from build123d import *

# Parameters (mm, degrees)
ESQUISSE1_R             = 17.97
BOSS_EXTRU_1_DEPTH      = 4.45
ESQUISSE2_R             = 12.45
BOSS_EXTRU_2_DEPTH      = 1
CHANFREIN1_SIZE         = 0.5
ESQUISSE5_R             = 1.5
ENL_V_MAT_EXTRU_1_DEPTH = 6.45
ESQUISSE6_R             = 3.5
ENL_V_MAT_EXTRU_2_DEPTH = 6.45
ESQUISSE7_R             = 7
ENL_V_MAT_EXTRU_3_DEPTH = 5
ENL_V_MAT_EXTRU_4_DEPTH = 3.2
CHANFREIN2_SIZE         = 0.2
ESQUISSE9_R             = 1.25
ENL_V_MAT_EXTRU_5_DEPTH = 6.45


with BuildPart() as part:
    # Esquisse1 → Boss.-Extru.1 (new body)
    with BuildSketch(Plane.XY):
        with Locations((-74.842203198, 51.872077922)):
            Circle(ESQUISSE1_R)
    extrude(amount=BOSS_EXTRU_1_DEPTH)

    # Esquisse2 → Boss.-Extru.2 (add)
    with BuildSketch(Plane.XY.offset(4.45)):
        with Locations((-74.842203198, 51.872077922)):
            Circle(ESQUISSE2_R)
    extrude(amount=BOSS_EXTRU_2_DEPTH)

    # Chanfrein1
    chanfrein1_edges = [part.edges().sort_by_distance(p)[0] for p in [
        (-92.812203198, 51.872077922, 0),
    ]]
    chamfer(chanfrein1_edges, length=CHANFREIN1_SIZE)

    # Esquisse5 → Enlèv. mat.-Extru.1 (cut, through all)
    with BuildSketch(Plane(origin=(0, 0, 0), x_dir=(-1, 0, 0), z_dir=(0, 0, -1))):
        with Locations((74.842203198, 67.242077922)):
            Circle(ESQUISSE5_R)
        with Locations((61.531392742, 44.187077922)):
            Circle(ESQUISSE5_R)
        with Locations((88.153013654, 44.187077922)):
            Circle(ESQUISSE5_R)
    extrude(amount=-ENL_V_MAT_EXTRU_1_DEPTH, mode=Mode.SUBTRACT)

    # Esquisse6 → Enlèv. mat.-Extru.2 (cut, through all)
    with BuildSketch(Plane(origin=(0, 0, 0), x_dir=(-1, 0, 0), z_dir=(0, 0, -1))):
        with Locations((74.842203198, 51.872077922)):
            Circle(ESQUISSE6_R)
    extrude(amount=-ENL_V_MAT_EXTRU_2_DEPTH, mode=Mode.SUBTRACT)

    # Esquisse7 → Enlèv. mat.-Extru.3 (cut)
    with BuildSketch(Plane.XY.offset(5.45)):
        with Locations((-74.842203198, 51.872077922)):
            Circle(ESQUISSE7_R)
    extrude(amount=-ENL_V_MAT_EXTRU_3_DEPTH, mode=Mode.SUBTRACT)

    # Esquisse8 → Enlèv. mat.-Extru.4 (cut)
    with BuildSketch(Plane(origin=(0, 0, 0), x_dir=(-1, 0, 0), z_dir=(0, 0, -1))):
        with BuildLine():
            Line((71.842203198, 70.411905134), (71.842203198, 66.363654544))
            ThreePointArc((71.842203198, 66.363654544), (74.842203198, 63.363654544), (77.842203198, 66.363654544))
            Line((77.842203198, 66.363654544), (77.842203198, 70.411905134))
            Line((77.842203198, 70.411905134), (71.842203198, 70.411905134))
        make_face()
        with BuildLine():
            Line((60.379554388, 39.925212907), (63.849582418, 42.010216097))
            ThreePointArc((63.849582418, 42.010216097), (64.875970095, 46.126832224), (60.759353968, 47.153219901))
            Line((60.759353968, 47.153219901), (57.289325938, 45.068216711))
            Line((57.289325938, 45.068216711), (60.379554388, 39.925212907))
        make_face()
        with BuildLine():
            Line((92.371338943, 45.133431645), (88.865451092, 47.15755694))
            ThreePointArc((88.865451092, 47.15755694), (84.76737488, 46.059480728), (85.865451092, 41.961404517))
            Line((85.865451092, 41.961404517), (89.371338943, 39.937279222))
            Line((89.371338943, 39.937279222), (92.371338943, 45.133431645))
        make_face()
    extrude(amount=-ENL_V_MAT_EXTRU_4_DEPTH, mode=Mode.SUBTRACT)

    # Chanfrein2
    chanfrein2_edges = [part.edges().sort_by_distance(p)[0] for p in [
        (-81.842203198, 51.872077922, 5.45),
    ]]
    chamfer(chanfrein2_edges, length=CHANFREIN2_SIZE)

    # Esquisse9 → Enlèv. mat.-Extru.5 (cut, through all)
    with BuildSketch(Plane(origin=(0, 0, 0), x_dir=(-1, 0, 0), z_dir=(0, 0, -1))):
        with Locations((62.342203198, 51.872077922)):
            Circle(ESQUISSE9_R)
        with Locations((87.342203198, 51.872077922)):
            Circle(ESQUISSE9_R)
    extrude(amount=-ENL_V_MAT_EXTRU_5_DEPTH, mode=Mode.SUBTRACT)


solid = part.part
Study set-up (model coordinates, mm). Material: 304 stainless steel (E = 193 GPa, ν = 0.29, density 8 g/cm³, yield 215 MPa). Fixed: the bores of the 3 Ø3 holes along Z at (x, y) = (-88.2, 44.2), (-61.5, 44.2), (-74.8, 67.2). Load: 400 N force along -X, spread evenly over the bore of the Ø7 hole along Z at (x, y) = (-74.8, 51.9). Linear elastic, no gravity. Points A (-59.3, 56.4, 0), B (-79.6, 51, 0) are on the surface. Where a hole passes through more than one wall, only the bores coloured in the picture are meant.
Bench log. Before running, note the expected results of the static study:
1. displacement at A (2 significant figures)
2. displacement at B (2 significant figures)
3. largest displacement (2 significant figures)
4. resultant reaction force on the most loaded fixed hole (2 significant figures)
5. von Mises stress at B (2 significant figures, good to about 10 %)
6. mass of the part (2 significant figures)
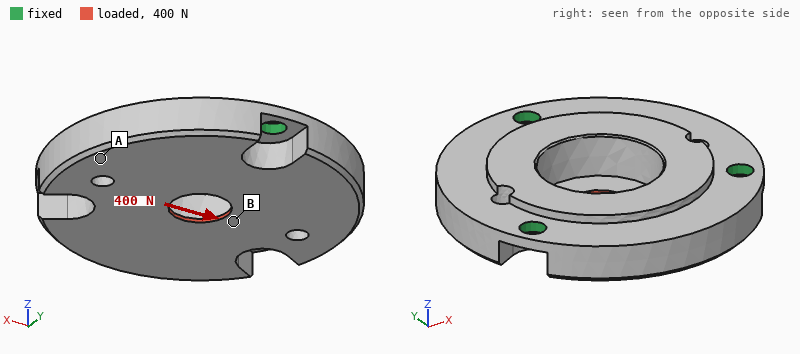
1.6 µm
1.5 µm
1.9 µm
150 N
37 MPa
30 g
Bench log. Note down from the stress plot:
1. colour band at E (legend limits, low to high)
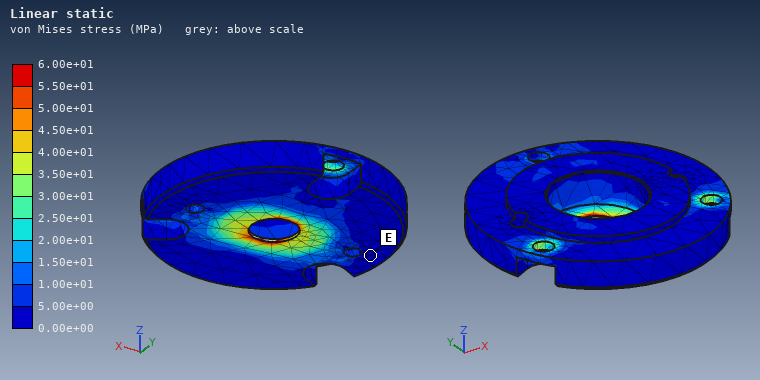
0.00e+00 to 5.00e+00 MPa
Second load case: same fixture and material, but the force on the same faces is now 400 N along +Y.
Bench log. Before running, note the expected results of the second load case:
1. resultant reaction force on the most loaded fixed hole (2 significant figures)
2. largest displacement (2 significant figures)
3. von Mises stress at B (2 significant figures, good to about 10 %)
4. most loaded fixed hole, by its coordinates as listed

170 N
2.1 µm
29 MPa
(-74.8, 67.2)
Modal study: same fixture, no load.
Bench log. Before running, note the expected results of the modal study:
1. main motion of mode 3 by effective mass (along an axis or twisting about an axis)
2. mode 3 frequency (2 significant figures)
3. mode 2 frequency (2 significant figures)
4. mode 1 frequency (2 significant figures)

along Z
16 kHz
13 kHz
13 kHz
